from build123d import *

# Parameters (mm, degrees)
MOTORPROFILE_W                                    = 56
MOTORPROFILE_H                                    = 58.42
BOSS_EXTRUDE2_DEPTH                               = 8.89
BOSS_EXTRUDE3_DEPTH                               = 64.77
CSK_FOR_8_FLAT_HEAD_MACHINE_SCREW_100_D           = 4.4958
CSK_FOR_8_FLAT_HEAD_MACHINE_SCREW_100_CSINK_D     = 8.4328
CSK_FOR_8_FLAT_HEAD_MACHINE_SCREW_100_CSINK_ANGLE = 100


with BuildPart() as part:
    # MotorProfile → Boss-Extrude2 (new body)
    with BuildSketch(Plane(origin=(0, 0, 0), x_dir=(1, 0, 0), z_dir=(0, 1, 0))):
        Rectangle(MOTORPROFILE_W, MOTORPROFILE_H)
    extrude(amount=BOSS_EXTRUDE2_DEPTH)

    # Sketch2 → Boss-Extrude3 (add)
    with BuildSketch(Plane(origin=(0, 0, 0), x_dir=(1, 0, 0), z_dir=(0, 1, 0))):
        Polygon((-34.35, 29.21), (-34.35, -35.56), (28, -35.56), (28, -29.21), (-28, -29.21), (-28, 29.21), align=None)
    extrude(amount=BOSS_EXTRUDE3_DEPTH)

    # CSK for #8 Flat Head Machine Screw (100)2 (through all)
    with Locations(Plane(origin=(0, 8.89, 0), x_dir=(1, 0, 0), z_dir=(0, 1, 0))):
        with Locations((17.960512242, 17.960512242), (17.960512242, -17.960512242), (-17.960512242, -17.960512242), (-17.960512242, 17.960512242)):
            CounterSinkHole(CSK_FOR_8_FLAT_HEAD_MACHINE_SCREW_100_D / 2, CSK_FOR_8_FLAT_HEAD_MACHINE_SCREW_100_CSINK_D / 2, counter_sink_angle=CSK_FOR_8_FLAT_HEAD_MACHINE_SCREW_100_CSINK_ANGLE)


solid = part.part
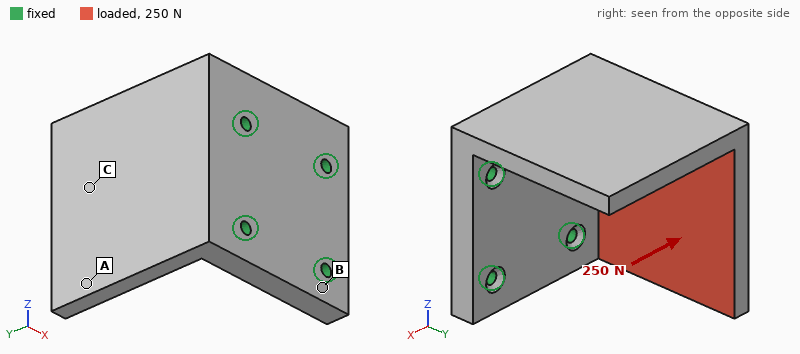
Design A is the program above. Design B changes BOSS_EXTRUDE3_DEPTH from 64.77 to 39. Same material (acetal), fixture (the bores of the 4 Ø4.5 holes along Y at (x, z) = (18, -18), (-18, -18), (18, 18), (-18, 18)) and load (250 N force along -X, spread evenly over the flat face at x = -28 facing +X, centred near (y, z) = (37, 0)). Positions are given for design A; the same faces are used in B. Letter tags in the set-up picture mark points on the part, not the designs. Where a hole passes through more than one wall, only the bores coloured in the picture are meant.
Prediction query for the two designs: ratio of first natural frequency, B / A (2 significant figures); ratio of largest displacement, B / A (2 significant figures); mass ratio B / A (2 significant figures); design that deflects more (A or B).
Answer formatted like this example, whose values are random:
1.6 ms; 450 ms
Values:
2.2; 0.39; 0.75; A
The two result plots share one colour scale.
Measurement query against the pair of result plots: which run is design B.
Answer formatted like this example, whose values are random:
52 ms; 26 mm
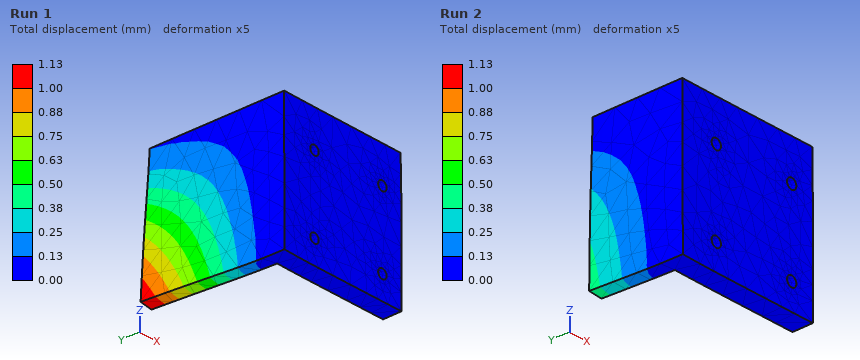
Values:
Run 2
